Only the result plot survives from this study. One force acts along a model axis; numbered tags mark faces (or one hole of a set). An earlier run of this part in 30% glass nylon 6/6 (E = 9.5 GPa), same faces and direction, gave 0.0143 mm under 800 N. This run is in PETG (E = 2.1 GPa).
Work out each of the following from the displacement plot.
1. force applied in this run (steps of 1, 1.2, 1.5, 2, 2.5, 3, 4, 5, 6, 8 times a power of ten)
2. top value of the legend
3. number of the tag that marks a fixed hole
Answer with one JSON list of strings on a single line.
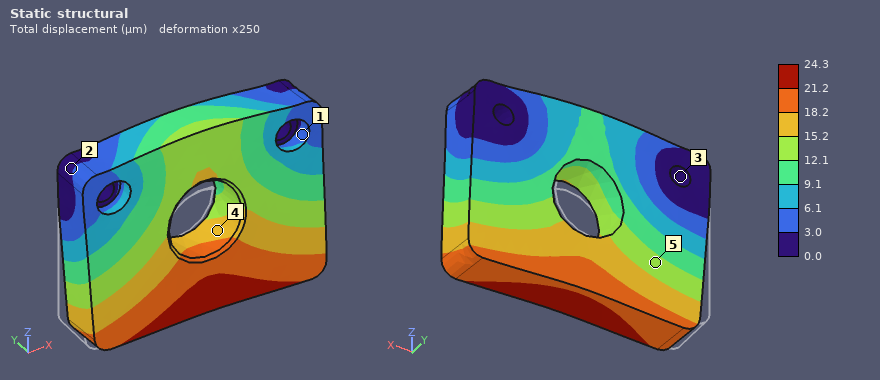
["300 N", "24.3 µm", "3"]
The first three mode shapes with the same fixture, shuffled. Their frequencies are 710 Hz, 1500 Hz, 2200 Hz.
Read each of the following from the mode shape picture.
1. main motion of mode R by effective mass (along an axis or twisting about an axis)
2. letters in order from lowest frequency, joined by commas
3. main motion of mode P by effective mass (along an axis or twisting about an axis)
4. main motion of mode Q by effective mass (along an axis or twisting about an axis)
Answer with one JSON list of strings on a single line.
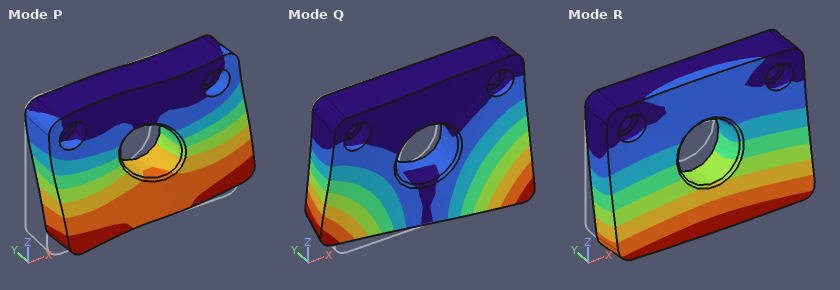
["along Y", "R, Q, P", "along X", "twisting about Z"]
